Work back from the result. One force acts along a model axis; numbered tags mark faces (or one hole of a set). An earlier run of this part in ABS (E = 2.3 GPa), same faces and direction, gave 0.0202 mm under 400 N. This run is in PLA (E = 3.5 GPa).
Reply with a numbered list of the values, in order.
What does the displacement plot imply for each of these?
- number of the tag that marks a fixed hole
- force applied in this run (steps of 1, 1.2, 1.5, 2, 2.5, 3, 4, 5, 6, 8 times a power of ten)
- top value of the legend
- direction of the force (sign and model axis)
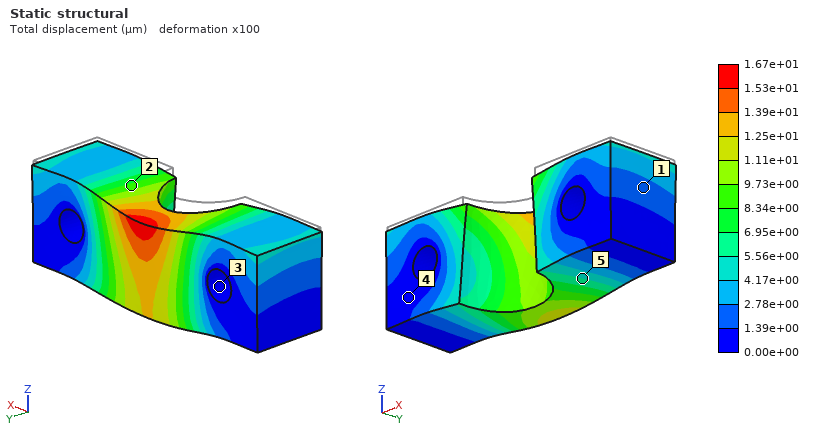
1. 3
2. 500 N
3. 1.67e+01 µm
4. -Z
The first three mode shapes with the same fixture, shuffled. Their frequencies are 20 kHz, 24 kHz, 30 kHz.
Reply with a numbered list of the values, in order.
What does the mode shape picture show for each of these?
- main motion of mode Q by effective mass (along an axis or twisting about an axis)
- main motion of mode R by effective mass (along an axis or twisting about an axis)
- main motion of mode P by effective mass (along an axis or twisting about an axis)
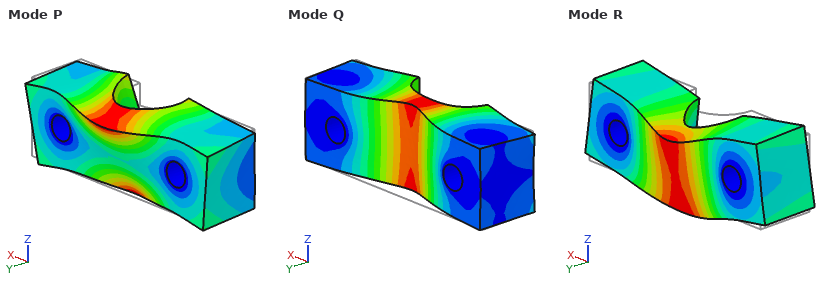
1. along Y
2. along Z
3. twisting about X
